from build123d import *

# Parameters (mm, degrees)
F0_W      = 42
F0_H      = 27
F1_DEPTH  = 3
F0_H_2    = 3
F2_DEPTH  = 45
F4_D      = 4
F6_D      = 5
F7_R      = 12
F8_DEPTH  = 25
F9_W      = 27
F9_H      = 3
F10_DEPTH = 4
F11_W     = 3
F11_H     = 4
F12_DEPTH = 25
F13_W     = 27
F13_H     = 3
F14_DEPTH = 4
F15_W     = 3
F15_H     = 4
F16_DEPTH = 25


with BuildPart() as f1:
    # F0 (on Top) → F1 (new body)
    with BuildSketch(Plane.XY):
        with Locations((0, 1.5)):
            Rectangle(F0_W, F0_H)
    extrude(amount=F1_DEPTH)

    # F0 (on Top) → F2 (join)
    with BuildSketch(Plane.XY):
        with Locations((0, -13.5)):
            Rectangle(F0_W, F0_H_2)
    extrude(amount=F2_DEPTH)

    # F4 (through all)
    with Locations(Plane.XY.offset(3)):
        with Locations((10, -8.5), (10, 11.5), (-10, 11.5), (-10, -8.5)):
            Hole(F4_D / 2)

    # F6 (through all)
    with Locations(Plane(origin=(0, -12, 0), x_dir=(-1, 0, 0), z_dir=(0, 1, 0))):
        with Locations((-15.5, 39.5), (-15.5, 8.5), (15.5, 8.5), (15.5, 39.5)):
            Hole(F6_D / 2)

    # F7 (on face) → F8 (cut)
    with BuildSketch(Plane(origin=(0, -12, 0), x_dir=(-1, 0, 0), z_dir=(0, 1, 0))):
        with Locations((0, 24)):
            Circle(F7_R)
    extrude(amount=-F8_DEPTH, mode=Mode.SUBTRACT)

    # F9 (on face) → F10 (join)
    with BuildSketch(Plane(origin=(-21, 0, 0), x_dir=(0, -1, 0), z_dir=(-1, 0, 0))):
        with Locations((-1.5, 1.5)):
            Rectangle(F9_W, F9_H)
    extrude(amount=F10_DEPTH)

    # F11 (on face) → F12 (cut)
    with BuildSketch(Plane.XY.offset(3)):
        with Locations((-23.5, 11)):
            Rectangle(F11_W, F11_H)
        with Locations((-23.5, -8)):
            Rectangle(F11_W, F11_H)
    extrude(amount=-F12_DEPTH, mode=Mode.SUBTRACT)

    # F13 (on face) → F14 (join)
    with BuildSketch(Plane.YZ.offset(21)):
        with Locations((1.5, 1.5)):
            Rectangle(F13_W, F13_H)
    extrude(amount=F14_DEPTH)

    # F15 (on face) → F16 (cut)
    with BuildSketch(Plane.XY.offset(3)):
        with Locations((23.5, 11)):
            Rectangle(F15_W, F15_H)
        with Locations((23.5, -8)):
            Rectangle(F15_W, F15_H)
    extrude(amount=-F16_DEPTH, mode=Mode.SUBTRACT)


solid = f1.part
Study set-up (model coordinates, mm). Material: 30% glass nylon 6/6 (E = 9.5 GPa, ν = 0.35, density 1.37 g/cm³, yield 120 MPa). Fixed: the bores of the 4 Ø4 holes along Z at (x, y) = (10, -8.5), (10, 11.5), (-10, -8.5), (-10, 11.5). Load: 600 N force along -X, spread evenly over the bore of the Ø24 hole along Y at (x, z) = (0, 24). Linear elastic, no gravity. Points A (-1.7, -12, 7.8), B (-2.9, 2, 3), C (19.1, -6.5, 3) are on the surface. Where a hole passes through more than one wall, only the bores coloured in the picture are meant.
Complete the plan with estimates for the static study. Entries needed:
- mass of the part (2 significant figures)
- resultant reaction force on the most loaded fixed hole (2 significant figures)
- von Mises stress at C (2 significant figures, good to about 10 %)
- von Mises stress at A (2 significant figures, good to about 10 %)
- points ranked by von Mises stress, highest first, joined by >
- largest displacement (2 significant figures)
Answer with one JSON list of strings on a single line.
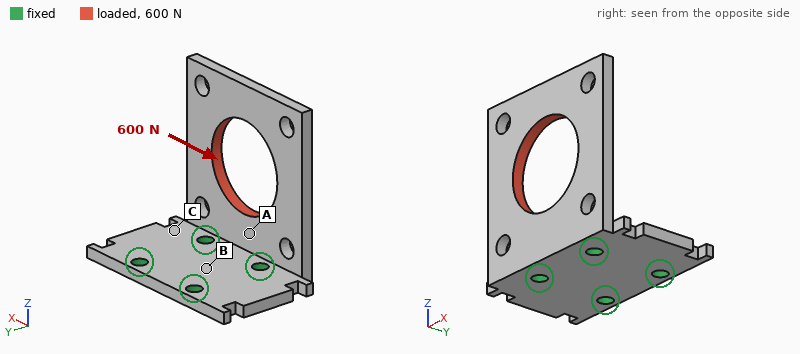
["11 g", "660 N", "24 MPa", "42 MPa", "A > C > B", "0.60 mm"]
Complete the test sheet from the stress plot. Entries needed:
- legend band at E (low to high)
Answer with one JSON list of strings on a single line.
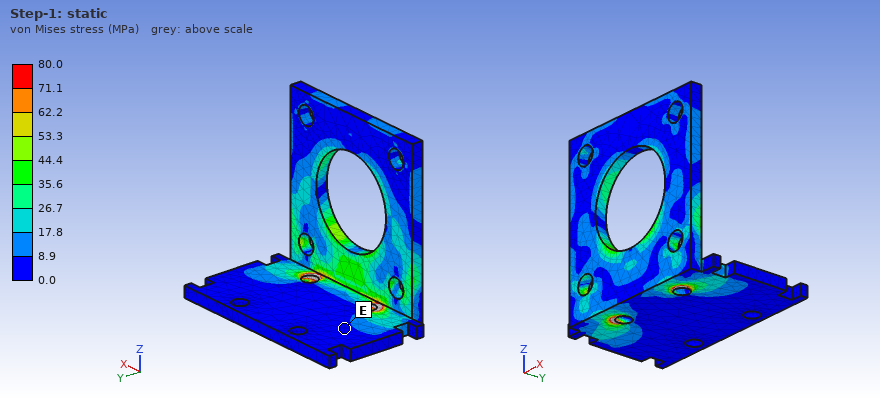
["0.0 to 8.9 MPa"]
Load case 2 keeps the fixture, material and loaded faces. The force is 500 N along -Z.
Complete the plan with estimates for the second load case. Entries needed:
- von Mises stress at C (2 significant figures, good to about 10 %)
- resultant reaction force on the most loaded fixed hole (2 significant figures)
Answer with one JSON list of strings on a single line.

["8.4 MPa", "260 N"]
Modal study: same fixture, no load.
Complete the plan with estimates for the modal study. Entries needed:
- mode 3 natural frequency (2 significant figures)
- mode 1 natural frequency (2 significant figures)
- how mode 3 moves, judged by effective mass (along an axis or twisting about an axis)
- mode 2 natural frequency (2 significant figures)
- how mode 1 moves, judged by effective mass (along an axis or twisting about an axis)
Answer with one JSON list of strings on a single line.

["2700 Hz", "550 Hz", "along X", "1300 Hz", "along Y"]
